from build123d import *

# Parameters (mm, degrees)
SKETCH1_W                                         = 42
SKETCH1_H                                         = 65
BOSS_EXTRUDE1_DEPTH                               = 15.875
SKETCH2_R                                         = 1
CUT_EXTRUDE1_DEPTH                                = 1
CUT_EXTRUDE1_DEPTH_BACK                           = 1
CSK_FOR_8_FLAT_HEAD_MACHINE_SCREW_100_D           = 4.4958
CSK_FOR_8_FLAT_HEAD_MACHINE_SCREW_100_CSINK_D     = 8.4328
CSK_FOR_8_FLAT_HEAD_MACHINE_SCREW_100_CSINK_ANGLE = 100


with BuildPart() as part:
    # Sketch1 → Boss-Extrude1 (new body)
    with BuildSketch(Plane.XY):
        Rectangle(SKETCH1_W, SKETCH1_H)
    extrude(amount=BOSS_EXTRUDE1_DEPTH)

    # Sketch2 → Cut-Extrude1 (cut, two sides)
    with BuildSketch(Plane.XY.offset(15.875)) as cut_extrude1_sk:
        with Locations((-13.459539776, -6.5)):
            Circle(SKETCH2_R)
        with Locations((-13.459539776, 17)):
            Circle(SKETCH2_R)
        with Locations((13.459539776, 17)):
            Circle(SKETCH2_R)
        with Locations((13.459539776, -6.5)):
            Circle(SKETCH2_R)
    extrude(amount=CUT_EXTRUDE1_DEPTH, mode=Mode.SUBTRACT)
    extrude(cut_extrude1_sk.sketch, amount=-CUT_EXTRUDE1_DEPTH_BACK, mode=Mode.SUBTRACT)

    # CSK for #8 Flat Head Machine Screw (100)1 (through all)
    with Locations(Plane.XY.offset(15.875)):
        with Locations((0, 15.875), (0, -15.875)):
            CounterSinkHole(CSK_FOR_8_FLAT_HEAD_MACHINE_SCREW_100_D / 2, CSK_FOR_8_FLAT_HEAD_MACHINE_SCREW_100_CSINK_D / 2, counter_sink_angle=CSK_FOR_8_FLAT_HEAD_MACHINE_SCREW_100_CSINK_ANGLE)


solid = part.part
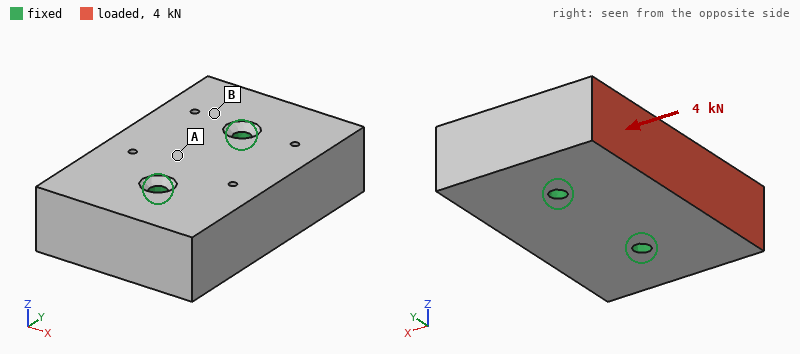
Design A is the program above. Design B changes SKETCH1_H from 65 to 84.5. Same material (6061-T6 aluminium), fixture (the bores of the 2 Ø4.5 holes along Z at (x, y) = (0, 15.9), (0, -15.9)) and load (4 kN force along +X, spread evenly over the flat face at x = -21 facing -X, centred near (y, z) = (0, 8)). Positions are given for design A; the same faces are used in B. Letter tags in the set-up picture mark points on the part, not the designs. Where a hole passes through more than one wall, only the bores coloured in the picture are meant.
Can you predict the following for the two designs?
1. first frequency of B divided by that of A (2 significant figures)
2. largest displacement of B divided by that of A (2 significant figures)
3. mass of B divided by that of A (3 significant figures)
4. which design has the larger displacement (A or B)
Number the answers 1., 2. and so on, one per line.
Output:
1. 0.83
2. 1.6
3. 1.30
4. B
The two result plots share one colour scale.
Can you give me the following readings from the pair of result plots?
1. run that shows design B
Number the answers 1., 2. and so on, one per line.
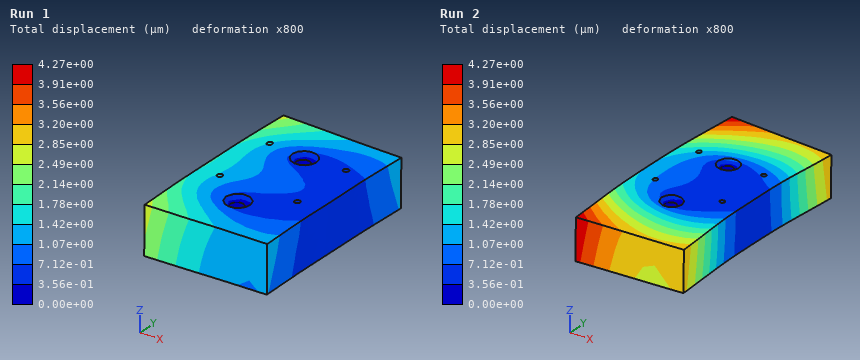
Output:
1. Run 2
